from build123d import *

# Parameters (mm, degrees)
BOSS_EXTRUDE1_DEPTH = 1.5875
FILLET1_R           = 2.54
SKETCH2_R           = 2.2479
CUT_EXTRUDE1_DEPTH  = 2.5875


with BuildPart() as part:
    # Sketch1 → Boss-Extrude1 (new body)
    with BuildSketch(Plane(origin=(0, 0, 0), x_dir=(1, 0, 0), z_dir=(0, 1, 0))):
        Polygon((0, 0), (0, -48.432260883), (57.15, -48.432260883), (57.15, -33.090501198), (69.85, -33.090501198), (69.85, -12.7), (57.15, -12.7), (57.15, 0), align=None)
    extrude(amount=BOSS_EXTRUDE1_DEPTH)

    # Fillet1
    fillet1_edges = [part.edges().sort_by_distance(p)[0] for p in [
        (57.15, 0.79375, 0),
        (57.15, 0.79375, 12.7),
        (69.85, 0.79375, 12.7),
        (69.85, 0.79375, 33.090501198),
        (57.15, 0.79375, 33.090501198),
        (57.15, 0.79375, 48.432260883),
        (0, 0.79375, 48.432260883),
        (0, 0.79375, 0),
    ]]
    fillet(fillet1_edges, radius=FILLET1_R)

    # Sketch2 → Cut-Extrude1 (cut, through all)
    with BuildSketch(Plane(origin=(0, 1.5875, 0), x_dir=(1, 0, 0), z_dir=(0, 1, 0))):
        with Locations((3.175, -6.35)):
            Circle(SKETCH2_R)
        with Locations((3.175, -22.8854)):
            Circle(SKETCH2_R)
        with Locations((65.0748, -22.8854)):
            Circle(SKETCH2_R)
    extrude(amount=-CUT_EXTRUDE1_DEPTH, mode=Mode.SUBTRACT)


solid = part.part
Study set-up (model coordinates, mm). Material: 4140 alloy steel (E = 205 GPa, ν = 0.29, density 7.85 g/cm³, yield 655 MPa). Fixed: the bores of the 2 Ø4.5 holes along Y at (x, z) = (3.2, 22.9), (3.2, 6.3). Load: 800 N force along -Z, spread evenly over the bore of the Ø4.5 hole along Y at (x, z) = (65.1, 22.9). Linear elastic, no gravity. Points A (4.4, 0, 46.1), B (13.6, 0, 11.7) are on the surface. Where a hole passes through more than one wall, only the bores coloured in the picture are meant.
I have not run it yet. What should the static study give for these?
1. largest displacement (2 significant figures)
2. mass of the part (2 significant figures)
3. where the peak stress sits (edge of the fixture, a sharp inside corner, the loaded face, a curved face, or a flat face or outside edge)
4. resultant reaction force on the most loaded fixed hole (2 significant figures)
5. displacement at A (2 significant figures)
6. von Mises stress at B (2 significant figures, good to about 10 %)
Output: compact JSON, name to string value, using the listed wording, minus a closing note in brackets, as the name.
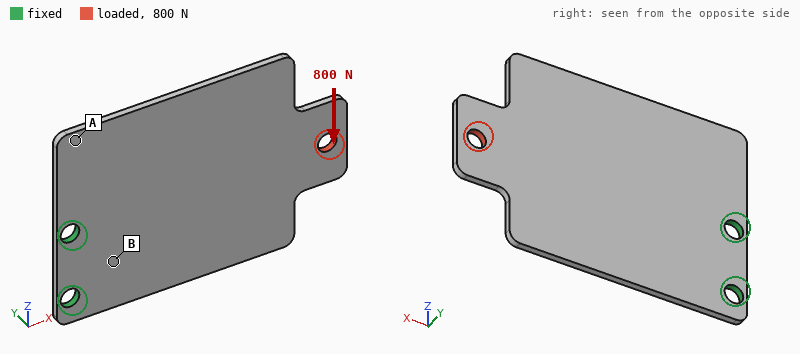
{"largest displacement": "94 µm", "mass of the part": "37 g", "where the peak stress sits": "edge of the fixture", "resultant reaction force on the most loaded fixed hole": "2.5 kN", "displacement at A": "34 µm", "von Mises stress at B": "91 MPa"}
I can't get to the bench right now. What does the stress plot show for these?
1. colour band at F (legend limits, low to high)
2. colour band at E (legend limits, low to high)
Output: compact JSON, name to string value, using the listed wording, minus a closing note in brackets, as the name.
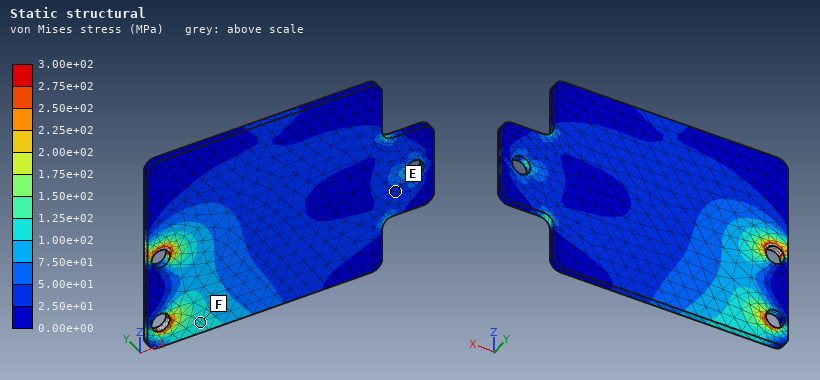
{"colour band at F": "1.00e+02 to 1.25e+02 MPa", "colour band at E": "2.50e+01 to 5.00e+01 MPa"}
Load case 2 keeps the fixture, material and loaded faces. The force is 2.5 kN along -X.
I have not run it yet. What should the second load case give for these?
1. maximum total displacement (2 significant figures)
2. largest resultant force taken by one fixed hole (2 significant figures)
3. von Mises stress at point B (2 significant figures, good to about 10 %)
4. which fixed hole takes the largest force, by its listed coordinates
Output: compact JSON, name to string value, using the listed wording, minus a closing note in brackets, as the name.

{"maximum total displacement": "38 µm", "largest resultant force taken by one fixed hole": "2.3 kN", "von Mises stress at point B": "37 MPa", "which fixed hole takes the largest force, by its listed coordinates": "(3.2, 22.9)"}
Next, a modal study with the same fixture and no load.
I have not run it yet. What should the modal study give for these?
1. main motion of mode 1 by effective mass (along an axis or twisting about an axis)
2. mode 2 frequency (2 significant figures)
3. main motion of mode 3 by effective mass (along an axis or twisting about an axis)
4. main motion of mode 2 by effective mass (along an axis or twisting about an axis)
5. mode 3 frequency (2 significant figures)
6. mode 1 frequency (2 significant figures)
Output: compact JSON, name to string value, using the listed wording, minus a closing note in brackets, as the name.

{"main motion of mode 1 by effective mass": "along Y", "mode 2 frequency": "980 Hz", "main motion of mode 3 by effective mass": "along Y", "main motion of mode 2 by effective mass": "twisting about X", "mode 3 frequency": "1900 Hz", "mode 1 frequency": "350 Hz"}
